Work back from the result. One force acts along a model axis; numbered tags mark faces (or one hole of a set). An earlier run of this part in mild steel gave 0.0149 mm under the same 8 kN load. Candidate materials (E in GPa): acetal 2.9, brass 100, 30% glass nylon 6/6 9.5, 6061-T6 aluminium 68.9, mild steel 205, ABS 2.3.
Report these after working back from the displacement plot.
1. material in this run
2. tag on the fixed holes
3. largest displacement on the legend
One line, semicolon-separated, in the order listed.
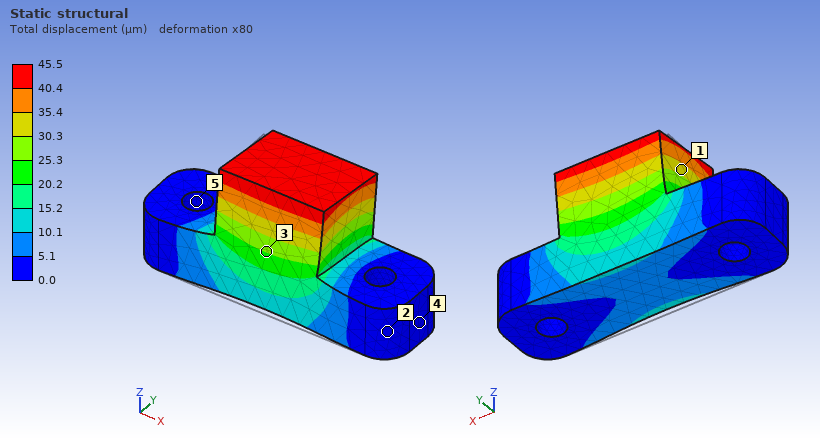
6061-T6 aluminium; 5; 45.5 µm
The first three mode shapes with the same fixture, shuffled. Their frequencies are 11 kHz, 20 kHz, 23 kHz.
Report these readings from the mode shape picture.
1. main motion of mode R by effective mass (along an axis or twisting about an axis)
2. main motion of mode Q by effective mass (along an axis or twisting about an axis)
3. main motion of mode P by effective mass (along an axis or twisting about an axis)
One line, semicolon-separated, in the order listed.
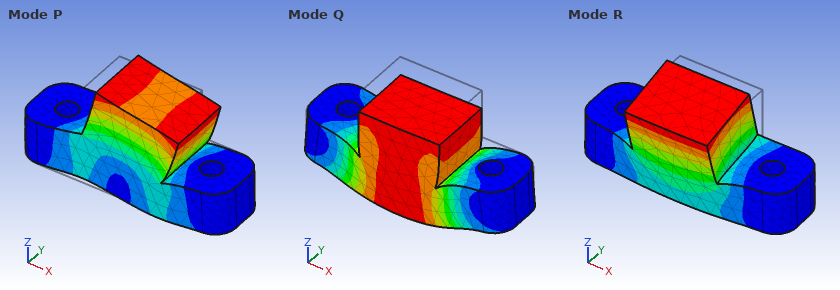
along Y; along Z; along X
